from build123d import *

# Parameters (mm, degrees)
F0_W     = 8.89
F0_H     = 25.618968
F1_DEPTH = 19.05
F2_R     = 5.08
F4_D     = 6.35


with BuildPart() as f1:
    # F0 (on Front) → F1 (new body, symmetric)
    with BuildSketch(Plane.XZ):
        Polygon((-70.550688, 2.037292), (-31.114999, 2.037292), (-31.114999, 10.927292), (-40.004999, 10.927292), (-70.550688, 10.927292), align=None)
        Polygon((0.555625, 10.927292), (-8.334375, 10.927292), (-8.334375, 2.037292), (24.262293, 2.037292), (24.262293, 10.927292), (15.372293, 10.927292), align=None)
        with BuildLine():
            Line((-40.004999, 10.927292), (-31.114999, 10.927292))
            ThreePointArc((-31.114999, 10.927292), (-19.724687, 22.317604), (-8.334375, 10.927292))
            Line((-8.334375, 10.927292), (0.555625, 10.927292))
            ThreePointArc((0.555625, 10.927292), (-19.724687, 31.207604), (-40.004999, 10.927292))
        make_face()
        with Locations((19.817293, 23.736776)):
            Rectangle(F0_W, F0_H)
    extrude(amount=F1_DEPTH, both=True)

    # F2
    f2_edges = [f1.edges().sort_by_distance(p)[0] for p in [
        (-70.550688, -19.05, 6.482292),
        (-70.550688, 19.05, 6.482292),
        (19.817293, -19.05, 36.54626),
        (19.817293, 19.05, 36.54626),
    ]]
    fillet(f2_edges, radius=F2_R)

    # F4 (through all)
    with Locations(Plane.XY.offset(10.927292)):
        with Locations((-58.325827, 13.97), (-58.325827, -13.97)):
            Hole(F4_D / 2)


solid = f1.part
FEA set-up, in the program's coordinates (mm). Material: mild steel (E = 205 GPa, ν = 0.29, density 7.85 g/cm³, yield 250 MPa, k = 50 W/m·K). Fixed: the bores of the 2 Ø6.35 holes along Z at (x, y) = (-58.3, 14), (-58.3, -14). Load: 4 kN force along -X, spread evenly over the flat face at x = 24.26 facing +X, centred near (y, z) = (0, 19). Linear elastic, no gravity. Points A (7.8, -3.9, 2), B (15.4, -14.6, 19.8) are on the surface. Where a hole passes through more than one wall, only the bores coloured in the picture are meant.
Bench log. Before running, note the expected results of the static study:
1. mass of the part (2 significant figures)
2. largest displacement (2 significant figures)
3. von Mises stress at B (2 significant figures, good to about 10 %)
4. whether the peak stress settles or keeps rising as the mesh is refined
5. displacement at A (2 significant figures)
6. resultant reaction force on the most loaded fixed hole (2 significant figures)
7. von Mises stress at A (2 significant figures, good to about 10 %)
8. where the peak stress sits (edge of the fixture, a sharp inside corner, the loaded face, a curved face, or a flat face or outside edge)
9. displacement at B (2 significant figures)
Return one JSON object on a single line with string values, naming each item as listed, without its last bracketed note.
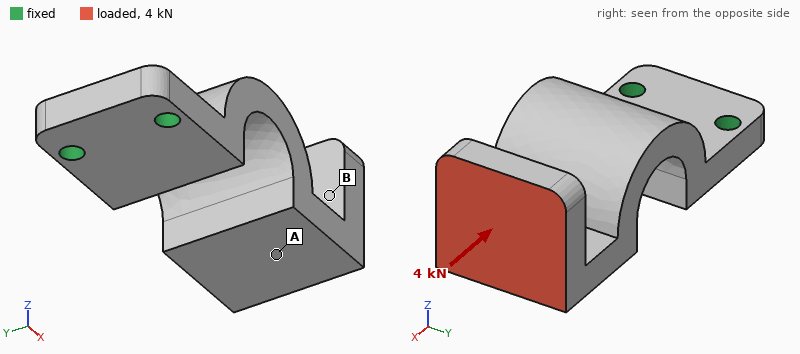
{"mass of the part": "390 g", "largest displacement": "0.25 mm", "von Mises stress at B": "29 MPa", "whether the peak stress settles or keeps rising as the mesh is refined": "keeps rising", "displacement at A": "0.12 mm", "resultant reaction force on the most loaded fixed hole": "2.0 kN", "von Mises stress at A": "79 MPa", "where the peak stress sits": "edge of the fixture", "displacement at B": "0.17 mm"}
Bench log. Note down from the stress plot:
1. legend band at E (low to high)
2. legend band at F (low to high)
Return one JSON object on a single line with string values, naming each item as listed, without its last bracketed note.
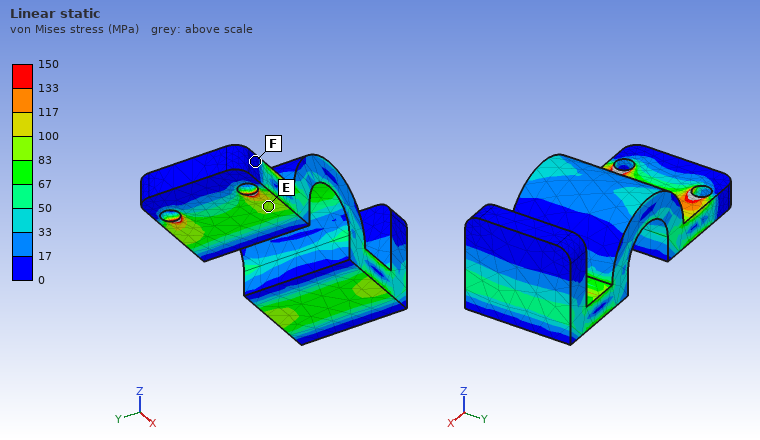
{"legend band at E": "83 to 100 MPa", "legend band at F": "0 to 17 MPa"}
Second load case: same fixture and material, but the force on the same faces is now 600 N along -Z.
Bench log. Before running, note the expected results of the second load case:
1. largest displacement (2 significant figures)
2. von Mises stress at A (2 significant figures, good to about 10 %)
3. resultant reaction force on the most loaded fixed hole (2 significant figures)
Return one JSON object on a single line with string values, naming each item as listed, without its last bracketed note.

{"largest displacement": "0.32 mm", "von Mises stress at A": "18 MPa", "resultant reaction force on the most loaded fixed hole": "310 N"}
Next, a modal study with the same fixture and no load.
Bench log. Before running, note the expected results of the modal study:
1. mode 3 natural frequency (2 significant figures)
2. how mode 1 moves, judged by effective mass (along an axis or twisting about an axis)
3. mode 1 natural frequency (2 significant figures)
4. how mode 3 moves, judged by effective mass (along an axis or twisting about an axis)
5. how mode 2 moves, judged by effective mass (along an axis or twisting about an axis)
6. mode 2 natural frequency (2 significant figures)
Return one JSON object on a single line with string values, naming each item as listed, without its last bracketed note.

{"mode 3 natural frequency": "2700 Hz", "how mode 1 moves, judged by effective mass": "along Z", "mode 1 natural frequency": "640 Hz", "how mode 3 moves, judged by effective mass": "along X", "how mode 2 moves, judged by effective mass": "along Y", "mode 2 natural frequency": "1500 Hz"}
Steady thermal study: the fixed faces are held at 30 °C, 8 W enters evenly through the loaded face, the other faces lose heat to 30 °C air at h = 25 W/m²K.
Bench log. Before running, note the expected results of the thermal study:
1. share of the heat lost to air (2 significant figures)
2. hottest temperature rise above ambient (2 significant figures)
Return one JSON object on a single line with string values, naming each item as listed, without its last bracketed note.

{"share of the heat lost to air": "53 %", "hottest temperature rise above ambient": "31 K"}
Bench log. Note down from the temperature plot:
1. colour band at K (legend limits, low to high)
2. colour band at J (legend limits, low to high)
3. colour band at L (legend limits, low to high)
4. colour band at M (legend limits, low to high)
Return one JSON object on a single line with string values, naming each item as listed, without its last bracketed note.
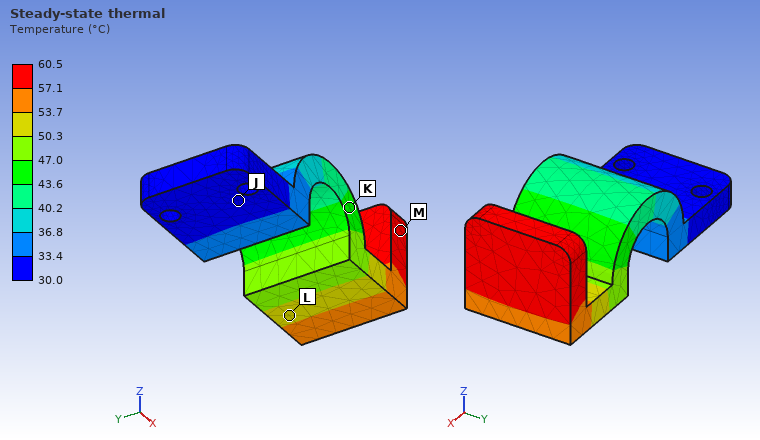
{"colour band at K": "43.6 to 47.0 °C", "colour band at J": "30.0 to 33.4 °C", "colour band at L": "50.3 to 53.7 °C", "colour band at M": "57.1 to 60.5 °C"}
